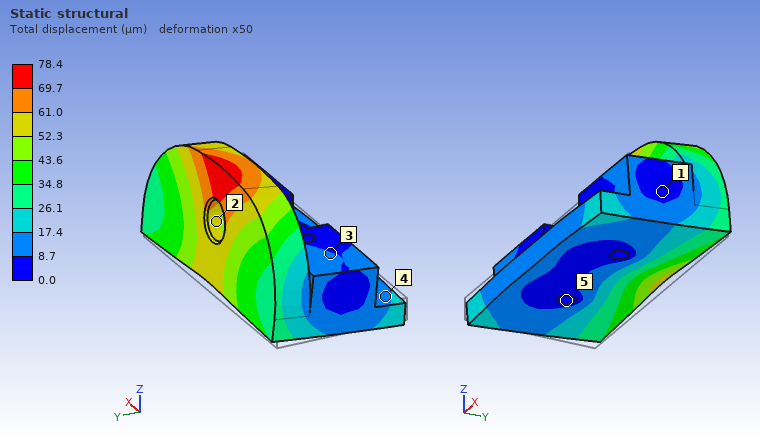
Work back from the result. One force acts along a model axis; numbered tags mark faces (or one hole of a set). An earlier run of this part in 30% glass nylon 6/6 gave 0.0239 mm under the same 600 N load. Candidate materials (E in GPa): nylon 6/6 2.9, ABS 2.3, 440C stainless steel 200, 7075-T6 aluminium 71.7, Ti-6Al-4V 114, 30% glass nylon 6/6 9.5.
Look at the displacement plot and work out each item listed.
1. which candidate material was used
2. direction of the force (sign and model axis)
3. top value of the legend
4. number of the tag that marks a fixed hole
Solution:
nylon 6/6
+Z
78.4 µm
5
